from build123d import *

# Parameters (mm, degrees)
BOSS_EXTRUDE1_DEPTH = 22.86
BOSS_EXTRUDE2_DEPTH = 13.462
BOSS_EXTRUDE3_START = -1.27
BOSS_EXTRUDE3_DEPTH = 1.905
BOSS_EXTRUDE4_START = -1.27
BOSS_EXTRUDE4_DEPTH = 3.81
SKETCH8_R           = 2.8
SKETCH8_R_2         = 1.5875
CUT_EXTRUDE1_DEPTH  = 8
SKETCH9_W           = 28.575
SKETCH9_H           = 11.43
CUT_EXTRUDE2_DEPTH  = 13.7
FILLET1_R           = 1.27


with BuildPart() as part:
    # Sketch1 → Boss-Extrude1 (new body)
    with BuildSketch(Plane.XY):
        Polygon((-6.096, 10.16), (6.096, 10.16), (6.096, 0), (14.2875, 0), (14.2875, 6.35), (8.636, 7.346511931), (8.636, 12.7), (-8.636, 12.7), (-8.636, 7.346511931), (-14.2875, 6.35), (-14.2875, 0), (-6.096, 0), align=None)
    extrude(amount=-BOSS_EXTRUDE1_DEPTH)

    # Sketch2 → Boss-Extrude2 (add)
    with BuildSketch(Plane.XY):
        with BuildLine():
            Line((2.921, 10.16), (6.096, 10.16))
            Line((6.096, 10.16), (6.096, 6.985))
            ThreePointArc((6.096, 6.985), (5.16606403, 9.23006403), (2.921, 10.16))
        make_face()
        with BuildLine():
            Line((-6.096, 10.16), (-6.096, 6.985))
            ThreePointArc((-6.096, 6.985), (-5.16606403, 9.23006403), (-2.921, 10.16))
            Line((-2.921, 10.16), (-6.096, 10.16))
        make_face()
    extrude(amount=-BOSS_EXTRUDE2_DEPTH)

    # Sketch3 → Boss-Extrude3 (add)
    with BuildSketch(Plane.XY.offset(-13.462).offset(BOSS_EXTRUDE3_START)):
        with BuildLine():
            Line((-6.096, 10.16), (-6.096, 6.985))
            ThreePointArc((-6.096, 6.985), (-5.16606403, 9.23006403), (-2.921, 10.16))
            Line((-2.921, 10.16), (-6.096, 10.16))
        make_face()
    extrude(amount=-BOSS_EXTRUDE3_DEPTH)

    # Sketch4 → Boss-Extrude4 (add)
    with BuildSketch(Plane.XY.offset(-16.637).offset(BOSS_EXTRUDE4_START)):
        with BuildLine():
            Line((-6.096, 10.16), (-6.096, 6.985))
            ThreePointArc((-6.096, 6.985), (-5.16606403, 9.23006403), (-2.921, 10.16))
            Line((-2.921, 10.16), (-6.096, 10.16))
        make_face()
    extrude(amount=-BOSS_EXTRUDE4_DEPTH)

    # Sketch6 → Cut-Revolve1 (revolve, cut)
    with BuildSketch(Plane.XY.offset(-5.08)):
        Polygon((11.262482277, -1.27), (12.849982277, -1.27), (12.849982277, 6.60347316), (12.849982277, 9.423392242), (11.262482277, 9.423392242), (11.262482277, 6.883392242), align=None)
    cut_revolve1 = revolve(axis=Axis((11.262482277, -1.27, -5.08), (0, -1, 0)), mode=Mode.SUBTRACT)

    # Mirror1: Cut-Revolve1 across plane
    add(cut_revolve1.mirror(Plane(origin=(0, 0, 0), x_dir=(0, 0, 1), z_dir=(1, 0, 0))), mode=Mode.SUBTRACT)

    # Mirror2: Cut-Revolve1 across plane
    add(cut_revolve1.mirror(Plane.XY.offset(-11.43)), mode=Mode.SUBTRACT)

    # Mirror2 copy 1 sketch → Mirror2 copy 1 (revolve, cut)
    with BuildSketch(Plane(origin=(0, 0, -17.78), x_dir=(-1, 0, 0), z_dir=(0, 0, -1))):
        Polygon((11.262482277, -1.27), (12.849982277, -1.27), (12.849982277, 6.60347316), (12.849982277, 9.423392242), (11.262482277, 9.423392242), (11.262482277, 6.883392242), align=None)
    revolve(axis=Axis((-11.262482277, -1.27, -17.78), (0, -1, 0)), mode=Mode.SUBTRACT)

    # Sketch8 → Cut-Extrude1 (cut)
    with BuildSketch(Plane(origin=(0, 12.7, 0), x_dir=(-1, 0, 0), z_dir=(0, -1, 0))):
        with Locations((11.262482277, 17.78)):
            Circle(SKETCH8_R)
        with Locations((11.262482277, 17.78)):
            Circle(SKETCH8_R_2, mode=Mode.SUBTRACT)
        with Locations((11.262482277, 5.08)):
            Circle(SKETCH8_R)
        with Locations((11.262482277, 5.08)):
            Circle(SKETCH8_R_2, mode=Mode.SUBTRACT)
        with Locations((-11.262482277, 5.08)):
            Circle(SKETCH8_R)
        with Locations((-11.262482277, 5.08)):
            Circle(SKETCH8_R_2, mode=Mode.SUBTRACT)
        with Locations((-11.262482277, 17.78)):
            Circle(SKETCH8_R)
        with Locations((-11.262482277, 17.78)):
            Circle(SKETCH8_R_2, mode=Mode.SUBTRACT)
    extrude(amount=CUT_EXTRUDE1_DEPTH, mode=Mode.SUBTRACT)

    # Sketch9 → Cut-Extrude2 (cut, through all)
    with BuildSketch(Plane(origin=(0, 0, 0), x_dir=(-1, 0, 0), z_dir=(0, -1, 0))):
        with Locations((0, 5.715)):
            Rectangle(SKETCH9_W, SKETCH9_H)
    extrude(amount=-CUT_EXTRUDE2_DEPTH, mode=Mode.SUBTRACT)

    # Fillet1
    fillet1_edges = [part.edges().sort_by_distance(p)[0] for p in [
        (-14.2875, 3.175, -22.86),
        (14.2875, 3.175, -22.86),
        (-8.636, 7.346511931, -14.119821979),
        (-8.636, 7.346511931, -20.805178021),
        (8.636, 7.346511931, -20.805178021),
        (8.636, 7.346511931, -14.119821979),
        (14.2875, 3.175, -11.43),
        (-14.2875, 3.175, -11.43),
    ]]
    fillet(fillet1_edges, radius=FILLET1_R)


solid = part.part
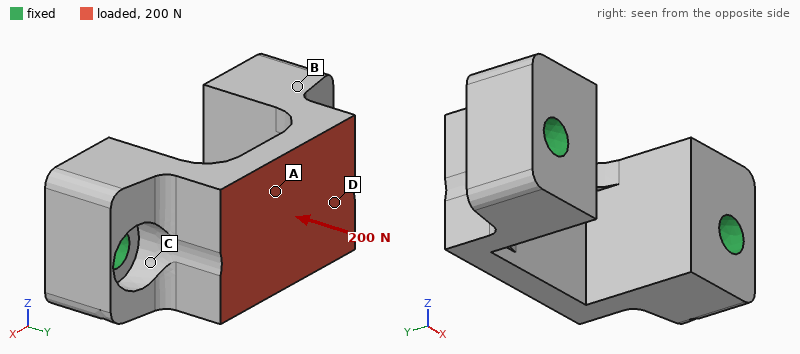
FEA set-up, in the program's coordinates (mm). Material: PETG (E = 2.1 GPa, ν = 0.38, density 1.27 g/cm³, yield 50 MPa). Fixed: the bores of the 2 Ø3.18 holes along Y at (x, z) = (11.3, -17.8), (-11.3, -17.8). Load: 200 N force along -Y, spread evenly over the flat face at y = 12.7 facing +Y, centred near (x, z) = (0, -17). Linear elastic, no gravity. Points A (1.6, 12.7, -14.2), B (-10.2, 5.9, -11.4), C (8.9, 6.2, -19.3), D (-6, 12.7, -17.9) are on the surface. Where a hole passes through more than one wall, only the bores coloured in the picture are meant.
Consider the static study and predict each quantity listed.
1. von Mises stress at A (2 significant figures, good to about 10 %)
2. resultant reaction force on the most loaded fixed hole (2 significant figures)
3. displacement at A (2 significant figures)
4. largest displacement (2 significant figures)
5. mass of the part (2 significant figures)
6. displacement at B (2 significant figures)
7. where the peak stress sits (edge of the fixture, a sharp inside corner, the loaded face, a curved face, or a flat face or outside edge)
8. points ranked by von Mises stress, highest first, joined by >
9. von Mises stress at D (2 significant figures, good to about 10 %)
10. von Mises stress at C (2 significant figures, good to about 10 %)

6.8 MPa
110 N
59 µm
71 µm
2.3 g
14 µm
a curved face
A > C > D > B
2.4 MPa
4.8 MPa
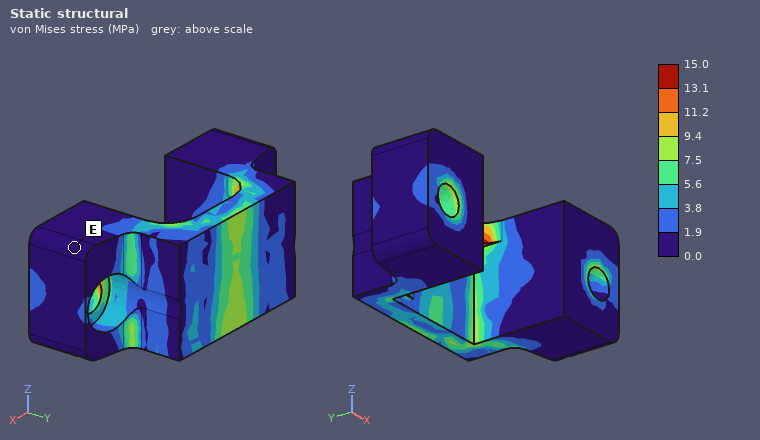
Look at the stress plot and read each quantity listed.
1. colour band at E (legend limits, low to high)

0.0 to 1.9 MPa
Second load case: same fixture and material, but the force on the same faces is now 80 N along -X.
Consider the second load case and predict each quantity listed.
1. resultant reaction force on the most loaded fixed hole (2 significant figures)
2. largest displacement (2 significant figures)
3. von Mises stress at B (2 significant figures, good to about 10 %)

47 N
53 µm
1.5 MPa
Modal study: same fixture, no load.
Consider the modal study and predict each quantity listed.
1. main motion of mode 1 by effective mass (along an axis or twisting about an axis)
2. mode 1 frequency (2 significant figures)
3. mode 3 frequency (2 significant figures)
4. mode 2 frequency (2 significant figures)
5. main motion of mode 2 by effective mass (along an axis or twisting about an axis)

along Z
5900 Hz
8800 Hz
7300 Hz
along X
